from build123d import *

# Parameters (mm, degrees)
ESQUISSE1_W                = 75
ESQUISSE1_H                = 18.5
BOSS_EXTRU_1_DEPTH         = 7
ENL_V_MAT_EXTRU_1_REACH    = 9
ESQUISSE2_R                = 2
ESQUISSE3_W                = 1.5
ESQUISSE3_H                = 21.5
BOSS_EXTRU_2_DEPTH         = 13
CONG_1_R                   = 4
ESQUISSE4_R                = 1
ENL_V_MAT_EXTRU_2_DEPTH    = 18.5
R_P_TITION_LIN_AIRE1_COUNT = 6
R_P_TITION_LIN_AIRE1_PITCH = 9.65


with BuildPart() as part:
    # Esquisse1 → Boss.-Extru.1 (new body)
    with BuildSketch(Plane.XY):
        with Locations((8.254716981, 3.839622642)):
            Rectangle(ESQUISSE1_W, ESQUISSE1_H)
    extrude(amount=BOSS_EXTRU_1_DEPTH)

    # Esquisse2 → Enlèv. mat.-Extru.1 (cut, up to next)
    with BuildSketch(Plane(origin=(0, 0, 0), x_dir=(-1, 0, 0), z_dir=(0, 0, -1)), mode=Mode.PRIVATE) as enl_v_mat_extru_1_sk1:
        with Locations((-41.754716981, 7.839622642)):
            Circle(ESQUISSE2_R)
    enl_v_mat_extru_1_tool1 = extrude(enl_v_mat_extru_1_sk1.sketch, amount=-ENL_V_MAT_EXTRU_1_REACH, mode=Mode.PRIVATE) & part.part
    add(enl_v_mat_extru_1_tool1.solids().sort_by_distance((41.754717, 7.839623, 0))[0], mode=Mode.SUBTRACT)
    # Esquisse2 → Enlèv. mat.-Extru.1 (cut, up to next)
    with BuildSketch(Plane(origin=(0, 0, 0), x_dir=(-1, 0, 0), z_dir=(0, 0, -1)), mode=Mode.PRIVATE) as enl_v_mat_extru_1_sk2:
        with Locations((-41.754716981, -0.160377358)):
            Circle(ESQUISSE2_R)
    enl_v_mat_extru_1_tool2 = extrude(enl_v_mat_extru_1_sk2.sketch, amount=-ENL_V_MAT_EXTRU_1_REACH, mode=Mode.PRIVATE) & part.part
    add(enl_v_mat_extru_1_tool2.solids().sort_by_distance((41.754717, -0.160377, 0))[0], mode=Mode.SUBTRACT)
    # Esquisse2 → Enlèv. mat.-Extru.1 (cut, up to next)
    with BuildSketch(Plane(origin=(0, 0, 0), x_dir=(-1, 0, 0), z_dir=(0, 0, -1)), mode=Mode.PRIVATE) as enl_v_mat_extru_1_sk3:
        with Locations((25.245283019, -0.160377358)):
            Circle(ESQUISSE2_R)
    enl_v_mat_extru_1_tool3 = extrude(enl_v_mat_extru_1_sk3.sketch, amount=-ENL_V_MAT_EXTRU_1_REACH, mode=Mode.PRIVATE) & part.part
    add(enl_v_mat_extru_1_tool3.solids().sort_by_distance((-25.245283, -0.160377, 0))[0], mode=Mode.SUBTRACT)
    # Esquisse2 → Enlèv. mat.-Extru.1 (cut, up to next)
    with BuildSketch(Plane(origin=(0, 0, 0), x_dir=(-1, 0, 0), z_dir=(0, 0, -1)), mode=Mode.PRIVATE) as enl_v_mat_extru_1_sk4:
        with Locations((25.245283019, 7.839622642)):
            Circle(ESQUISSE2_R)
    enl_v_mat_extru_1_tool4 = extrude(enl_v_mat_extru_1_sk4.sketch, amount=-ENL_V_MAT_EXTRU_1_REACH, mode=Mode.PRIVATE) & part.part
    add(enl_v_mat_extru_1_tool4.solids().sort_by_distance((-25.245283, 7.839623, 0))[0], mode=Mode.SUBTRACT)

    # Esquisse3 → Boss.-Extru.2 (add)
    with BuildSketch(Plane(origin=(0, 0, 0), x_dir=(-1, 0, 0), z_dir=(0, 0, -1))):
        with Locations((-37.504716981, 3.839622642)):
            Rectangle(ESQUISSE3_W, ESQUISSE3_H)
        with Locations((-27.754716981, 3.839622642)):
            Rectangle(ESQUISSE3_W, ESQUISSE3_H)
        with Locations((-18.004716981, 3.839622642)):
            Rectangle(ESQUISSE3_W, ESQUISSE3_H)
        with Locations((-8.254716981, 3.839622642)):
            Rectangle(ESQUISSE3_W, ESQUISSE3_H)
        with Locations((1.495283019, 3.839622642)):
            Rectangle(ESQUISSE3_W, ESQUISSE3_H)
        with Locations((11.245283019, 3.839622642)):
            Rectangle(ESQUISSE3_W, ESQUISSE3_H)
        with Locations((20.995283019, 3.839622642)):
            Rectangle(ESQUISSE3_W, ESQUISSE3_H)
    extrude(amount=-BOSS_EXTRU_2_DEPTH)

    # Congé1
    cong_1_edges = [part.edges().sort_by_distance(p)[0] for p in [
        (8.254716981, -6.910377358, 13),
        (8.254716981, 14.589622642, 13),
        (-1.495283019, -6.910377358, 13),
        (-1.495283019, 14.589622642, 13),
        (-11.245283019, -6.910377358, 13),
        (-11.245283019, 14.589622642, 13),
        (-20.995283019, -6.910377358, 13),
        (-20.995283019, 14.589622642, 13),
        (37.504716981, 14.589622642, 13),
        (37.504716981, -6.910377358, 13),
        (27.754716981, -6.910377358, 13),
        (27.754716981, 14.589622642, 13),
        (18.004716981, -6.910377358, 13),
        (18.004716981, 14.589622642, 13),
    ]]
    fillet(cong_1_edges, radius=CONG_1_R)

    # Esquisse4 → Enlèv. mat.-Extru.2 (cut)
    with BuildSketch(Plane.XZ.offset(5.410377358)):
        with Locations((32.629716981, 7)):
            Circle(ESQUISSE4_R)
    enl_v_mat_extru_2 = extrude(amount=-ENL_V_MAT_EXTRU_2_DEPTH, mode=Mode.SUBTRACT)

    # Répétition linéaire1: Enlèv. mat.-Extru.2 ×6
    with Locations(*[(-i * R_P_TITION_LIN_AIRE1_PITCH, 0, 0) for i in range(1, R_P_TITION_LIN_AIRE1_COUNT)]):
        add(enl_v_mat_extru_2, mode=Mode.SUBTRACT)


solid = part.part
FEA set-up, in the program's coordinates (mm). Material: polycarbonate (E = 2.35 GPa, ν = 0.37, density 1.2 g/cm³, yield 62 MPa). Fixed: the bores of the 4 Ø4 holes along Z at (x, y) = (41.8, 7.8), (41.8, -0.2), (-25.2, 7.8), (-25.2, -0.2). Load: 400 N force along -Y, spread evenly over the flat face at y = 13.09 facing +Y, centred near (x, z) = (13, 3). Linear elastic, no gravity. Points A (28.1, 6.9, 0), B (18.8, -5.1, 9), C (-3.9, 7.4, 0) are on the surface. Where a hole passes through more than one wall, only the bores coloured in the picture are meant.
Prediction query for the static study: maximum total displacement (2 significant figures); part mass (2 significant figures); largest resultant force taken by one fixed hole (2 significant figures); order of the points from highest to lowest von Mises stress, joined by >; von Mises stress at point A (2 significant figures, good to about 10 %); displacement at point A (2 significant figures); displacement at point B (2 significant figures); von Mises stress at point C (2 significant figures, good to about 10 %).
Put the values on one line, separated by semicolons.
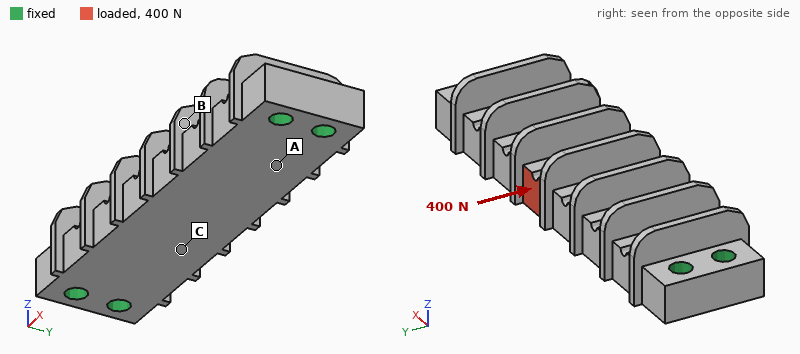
0.15 mm; 13 g; 310 N; A > C > B; 4.5 MPa; 0.064 mm; 0.12 mm; 3.0 MPa
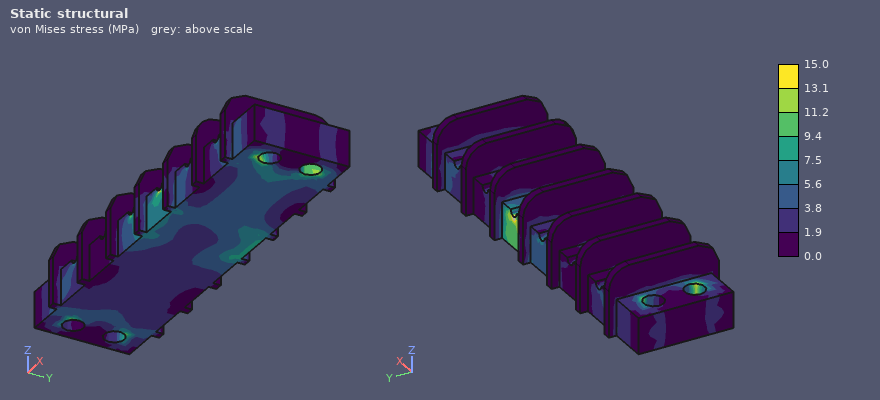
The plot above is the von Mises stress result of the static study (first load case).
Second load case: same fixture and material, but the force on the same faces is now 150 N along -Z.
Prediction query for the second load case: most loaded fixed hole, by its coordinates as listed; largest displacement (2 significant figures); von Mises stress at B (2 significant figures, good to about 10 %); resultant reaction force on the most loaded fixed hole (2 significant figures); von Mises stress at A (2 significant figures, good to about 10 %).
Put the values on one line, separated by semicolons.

(41.8, 7.8); 0.35 mm; 1.6 MPa; 96 N; 6.1 MPa
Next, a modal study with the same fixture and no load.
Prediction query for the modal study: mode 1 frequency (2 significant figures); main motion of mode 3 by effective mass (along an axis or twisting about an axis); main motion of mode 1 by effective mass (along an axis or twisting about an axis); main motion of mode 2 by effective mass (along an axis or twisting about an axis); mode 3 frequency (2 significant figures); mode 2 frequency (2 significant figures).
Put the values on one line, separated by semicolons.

2000 Hz; along Y; along Z; along Y; 3900 Hz; 3400 Hz
